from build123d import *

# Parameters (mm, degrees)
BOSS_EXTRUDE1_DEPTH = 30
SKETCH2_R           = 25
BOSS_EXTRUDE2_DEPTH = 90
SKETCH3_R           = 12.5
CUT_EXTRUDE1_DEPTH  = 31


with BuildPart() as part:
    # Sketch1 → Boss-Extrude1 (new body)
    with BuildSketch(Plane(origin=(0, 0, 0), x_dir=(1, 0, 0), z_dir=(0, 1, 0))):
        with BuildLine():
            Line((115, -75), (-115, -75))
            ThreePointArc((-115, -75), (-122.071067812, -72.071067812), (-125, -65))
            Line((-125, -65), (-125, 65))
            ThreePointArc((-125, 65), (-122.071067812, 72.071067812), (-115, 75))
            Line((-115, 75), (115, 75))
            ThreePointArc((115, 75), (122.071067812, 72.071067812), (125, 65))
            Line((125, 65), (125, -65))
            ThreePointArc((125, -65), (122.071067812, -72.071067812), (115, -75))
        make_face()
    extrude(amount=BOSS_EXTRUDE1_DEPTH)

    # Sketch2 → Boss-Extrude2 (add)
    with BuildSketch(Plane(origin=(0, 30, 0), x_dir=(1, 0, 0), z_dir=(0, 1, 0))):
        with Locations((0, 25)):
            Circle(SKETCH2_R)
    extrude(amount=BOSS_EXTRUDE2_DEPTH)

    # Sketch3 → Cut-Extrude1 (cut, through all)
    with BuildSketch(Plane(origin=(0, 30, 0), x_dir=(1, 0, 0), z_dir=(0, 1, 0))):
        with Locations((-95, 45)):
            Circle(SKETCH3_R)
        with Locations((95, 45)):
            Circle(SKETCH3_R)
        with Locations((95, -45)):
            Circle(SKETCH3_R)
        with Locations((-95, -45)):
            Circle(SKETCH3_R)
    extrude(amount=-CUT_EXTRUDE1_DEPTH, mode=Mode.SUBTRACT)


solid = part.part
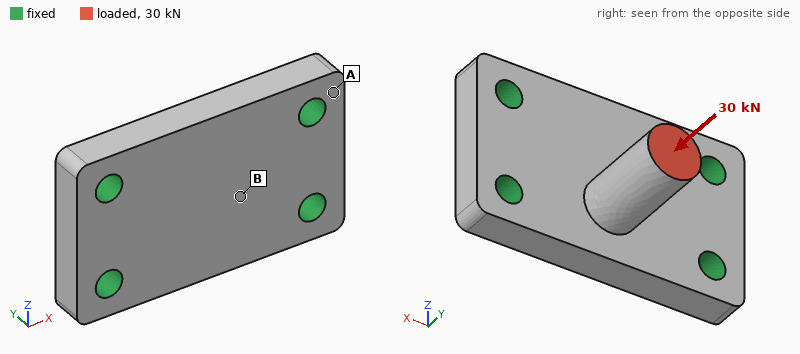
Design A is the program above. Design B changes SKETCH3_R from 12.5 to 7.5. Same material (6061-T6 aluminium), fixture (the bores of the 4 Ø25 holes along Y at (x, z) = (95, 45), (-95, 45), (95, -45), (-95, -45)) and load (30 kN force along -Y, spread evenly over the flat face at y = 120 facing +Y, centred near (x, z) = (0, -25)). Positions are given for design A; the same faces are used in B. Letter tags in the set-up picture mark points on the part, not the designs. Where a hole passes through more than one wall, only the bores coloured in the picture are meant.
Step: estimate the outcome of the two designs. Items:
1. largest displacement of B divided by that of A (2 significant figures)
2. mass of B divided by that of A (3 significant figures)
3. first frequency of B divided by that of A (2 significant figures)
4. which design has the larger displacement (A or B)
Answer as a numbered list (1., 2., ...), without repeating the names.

1. 1.2
2. 1.03
3. 0.97
4. B
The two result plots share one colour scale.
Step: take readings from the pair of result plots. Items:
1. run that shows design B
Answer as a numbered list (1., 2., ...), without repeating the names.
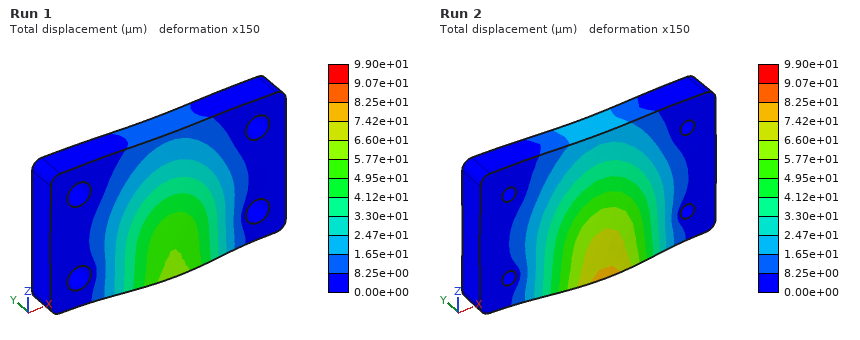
1. Run 2
